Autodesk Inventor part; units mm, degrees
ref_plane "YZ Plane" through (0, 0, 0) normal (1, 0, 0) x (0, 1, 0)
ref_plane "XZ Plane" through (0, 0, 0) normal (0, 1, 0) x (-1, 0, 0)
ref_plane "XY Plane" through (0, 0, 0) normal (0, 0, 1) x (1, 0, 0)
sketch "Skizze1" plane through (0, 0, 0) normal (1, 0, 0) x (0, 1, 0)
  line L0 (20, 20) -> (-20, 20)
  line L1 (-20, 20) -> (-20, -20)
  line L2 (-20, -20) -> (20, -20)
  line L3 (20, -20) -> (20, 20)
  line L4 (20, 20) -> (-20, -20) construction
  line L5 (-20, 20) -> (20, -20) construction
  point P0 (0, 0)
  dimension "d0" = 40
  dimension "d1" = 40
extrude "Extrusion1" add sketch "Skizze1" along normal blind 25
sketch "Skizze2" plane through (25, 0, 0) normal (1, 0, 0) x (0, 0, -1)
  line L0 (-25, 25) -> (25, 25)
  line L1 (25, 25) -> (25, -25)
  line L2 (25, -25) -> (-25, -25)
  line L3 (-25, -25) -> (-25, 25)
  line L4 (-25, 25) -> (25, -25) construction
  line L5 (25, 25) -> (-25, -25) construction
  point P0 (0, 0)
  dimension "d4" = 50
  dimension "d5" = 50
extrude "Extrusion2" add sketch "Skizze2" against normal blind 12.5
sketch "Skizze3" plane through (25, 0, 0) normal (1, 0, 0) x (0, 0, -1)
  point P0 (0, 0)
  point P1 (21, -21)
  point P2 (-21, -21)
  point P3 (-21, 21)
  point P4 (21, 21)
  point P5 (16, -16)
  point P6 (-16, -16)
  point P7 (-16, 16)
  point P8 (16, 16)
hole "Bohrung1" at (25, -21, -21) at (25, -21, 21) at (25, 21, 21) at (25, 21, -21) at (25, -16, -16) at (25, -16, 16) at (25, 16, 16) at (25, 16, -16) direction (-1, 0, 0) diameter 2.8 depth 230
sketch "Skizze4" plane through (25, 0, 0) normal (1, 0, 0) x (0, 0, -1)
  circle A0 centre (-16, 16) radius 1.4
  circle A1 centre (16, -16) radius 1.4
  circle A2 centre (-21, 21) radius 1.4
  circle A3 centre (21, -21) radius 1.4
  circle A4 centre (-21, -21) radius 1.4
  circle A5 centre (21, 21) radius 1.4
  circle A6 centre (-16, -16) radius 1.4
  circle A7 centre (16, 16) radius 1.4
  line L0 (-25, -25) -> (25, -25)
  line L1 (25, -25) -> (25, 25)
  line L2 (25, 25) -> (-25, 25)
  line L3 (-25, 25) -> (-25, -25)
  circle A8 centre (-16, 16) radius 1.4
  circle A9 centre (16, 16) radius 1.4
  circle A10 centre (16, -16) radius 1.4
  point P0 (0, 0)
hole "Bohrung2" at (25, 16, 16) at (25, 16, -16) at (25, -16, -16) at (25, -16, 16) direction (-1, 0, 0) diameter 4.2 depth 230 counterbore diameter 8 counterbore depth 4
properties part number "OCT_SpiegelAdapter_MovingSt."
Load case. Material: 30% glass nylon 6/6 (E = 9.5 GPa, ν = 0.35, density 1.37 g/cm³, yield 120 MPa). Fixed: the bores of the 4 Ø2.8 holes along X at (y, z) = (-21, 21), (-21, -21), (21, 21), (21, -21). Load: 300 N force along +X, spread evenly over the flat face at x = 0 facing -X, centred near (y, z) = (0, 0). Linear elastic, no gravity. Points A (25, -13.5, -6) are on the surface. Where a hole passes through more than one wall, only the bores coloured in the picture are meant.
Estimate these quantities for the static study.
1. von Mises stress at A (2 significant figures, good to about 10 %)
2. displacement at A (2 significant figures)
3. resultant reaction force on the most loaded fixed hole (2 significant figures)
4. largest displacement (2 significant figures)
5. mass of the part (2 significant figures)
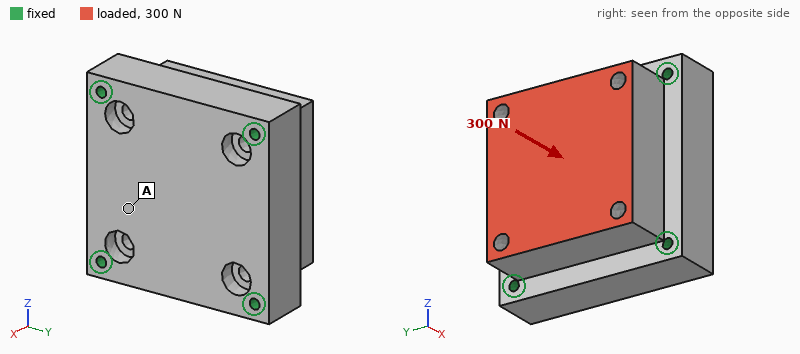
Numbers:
0.27 MPa
2.0 µm
78 N
2.4 µm
67 g
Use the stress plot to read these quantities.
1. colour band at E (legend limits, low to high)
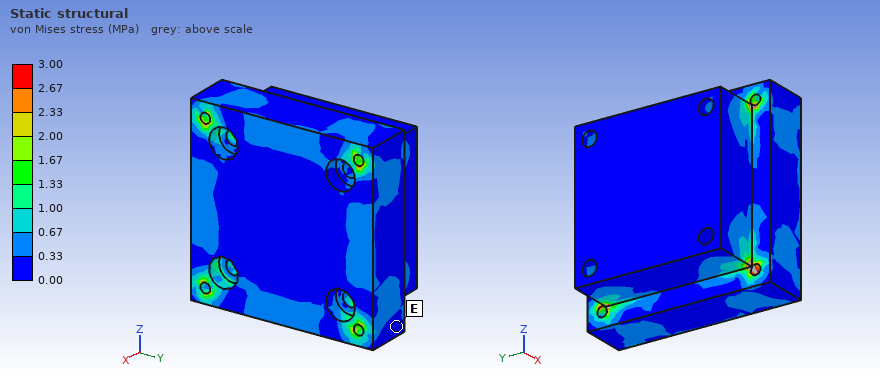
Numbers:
0.00 to 0.33 MPa
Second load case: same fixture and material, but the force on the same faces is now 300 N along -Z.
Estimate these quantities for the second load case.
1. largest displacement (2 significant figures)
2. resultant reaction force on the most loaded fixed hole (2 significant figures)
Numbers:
4.1 µm
100 N
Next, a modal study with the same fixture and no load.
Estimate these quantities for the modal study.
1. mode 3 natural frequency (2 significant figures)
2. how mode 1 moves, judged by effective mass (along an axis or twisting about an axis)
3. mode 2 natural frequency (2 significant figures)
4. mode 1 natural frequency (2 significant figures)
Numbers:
9500 Hz
along X
9500 Hz
7800 Hz
